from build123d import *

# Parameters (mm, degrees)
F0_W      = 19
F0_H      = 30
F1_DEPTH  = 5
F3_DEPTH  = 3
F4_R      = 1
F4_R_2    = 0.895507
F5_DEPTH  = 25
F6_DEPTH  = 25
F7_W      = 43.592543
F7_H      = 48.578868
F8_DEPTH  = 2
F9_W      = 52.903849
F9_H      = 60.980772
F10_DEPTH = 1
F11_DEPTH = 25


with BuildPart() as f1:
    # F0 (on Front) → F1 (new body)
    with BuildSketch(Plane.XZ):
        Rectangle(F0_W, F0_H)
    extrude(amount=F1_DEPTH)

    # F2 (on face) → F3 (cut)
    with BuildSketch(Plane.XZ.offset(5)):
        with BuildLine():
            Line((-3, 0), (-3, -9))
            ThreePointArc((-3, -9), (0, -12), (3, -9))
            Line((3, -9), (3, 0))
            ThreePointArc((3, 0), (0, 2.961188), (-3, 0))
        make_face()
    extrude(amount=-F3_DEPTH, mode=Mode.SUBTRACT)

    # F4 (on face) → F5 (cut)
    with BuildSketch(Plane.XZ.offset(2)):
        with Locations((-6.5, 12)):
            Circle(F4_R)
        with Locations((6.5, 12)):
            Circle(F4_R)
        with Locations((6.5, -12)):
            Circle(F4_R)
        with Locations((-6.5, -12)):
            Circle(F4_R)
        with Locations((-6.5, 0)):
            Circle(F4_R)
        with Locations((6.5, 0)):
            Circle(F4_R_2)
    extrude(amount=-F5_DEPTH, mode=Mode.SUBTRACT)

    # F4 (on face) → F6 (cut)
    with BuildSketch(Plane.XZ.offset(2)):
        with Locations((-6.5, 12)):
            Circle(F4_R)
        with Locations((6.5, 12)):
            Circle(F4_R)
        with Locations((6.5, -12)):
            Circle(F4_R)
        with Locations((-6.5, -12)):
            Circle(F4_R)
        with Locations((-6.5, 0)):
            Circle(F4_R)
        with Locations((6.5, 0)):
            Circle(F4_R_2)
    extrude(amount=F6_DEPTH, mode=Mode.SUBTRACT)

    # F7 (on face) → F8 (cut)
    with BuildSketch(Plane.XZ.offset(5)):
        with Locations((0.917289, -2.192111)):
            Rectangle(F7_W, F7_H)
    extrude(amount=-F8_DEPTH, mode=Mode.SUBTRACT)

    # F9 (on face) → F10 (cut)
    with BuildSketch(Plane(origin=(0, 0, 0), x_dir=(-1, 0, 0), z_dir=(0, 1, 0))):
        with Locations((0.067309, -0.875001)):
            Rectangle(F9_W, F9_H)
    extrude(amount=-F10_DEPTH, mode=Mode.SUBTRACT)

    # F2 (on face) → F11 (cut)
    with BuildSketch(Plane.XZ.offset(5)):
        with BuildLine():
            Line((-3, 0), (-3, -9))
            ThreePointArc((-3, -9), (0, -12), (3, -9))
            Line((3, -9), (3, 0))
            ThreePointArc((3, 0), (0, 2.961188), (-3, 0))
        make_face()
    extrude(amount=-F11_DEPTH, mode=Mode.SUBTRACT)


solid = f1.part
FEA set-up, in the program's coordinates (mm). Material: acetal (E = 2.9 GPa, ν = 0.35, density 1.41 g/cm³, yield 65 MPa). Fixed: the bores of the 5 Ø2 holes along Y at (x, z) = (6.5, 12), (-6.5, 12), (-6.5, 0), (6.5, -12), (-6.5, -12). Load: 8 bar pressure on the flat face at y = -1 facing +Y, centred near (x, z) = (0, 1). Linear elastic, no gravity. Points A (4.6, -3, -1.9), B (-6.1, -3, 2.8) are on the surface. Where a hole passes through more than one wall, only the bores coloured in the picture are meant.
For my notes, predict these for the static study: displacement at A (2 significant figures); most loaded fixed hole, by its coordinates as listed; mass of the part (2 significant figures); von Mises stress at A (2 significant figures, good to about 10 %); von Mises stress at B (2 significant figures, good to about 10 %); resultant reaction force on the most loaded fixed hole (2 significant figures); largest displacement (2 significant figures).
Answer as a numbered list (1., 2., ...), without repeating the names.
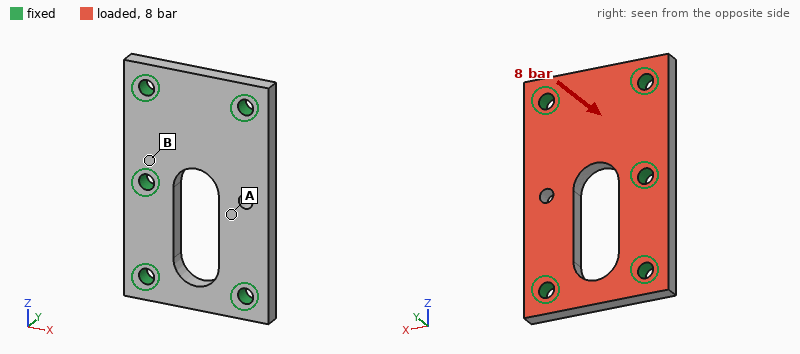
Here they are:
1. 0.28 mm
2. (6.5, 12)
3. 1.3 g
4. 23 MPa
5. 10 MPa
6. 98 N
7. 0.34 mm
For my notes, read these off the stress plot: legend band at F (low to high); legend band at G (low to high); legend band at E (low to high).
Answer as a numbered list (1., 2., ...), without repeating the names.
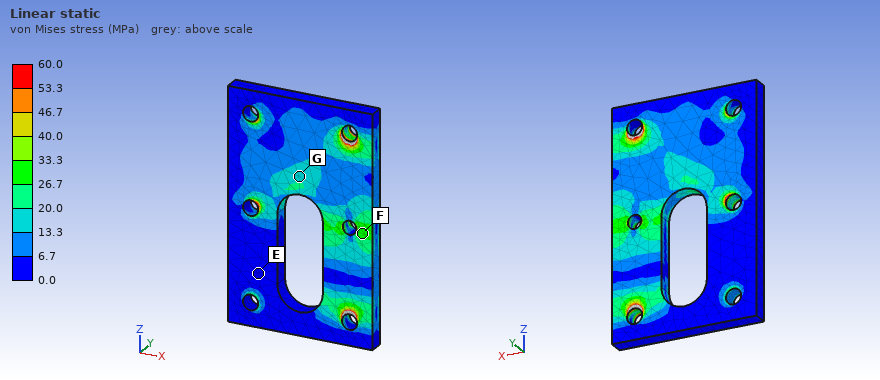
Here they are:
1. 26.7 to 33.3 MPa
2. 13.3 to 20.0 MPa
3. 0.0 to 6.7 MPa
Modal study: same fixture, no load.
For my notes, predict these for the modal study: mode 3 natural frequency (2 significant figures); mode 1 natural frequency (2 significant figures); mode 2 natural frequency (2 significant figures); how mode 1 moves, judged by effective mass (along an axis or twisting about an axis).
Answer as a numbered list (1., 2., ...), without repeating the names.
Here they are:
1. 13 kHz
2. 5700 Hz
3. 12 kHz
4. along Y
